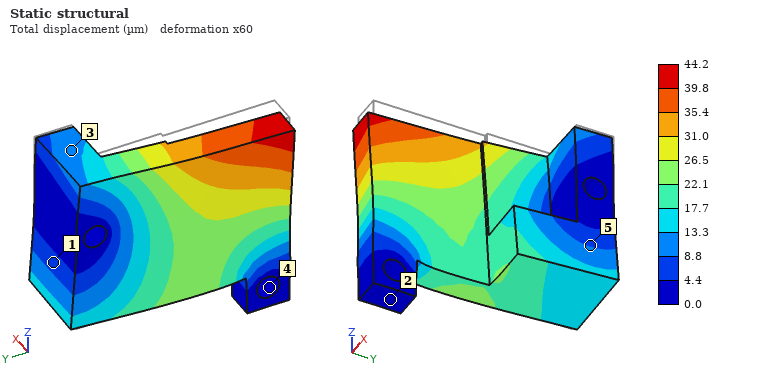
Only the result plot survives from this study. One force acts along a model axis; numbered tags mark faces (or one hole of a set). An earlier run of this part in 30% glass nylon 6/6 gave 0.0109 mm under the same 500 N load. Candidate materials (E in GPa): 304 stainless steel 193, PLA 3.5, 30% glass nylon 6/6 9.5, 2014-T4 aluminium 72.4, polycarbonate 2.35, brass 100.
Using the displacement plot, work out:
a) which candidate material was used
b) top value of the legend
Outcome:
polycarbonate
44.2 µm
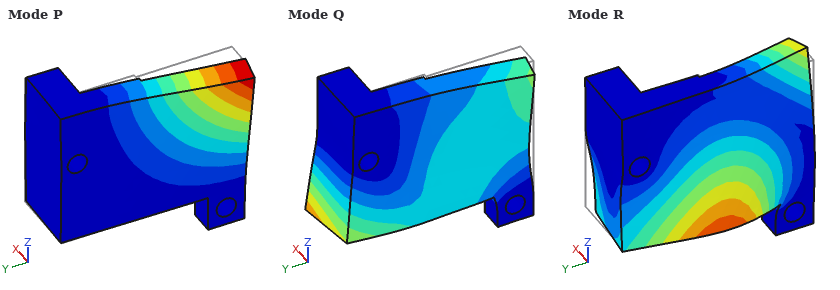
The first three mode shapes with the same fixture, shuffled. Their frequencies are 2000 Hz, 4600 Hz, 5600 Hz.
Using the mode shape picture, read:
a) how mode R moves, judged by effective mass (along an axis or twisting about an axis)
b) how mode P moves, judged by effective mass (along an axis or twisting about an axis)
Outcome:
along X
along X
